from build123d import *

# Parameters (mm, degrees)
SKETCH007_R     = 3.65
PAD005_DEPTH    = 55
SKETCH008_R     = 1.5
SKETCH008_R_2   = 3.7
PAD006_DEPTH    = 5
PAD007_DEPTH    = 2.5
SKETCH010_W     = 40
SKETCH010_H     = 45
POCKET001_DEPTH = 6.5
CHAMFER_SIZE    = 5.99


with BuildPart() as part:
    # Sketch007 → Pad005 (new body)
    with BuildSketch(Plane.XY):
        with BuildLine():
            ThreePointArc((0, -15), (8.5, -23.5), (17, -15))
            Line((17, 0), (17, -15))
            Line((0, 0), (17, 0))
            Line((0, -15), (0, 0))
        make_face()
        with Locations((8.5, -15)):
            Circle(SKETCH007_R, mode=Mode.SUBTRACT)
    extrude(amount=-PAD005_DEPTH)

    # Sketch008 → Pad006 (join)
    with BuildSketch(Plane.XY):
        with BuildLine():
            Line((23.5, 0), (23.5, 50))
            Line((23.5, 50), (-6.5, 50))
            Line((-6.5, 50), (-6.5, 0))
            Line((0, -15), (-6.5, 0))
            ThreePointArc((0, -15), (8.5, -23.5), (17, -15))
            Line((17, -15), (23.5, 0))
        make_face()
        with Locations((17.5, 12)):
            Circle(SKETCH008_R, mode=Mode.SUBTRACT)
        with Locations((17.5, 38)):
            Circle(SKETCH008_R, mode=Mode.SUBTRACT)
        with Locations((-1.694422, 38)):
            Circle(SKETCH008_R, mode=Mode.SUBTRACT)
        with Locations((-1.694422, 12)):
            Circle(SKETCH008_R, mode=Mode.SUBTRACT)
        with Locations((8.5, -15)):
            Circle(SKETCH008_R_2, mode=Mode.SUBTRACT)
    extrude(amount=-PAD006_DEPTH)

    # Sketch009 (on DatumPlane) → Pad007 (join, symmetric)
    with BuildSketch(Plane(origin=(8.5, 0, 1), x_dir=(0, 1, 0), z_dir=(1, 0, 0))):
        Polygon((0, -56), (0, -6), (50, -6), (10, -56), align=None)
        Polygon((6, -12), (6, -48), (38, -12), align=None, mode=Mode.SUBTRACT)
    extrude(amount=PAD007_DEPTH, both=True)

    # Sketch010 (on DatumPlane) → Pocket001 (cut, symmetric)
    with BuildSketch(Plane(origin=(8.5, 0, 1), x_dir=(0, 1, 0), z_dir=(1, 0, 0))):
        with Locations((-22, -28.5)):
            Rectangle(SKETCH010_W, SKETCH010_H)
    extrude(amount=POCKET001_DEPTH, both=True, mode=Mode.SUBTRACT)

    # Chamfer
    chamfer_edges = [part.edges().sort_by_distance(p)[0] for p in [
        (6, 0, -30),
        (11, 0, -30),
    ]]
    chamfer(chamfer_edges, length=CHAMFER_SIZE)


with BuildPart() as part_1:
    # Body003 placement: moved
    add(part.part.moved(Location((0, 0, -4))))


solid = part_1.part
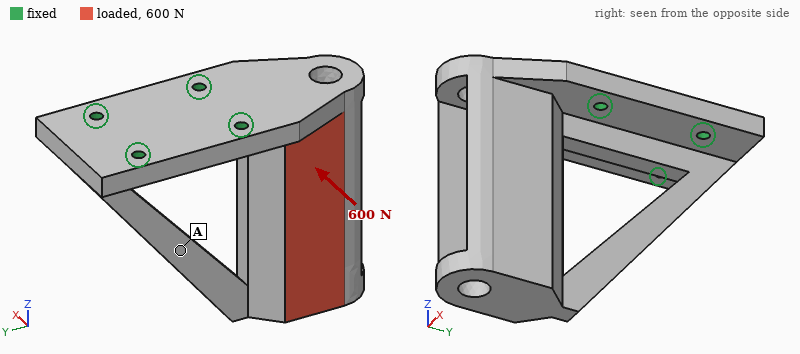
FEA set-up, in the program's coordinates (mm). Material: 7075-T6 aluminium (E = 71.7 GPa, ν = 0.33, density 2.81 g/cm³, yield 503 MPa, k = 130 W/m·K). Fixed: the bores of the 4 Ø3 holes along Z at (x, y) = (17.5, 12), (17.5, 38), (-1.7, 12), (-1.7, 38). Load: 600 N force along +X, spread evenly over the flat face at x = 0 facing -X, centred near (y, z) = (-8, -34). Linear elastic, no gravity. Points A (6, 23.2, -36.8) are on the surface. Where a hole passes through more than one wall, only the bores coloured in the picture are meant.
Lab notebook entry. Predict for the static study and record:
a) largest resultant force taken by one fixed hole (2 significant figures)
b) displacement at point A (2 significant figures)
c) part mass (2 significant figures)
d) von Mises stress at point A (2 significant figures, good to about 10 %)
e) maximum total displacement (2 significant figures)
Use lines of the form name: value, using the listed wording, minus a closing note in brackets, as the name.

largest resultant force taken by one fixed hole: 1.0 kN
displacement at point A: 0.048 mm
part mass: 62 g
von Mises stress at point A: 13 MPa
maximum total displacement: 0.24 mm
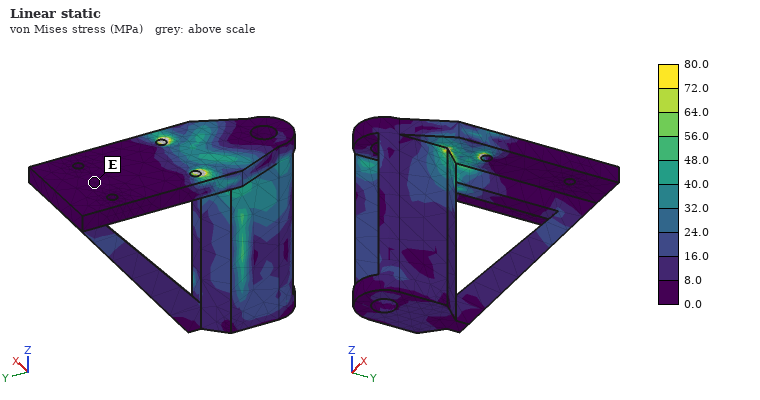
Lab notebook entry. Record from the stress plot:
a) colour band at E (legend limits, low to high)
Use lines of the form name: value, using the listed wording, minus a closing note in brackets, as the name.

colour band at E: 0.0 to 8.0 MPa
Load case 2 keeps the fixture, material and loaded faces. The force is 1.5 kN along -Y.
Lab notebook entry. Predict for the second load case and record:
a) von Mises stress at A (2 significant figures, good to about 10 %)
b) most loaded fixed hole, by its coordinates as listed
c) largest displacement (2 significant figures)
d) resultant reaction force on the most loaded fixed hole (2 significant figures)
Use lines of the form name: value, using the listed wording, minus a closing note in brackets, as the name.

von Mises stress at A: 47 MPa
most loaded fixed hole, by its coordinates as listed: (-1.7, 12)
largest displacement: 0.19 mm
resultant reaction force on the most loaded fixed hole: 1.0 kN
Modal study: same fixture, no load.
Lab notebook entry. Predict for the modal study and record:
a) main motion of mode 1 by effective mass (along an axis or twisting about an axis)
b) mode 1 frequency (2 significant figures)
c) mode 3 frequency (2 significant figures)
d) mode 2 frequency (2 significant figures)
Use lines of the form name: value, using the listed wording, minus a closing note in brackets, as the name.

main motion of mode 1 by effective mass: along X
mode 1 frequency: 1900 Hz
mode 3 frequency: 4300 Hz
mode 2 frequency: 3400 Hz
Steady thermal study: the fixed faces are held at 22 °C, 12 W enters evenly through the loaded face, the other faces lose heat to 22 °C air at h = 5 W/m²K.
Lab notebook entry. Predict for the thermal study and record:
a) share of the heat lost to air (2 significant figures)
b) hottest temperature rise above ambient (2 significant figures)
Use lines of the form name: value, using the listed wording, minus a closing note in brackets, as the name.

share of the heat lost to air: 4.3 %
hottest temperature rise above ambient: 20 K
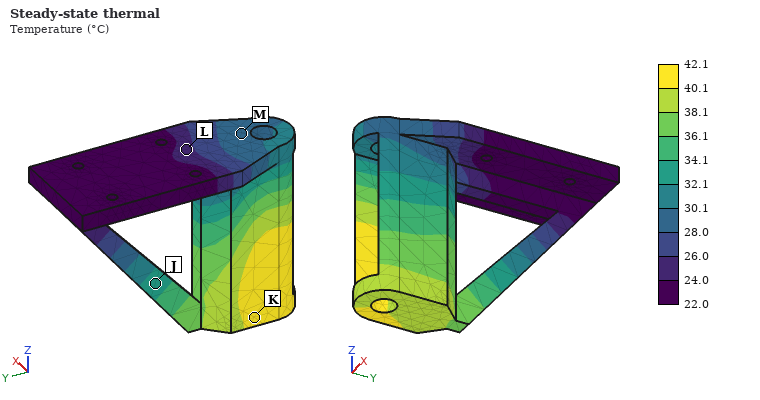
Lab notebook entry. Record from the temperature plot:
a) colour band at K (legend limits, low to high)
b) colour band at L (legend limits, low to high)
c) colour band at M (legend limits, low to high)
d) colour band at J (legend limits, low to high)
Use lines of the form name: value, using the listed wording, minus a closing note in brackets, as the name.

colour band at K: 40.1 to 42.1 °C
colour band at L: 24.0 to 26.0 °C
colour band at M: 28.0 to 30.1 °C
colour band at J: 32.1 to 34.1 °C
